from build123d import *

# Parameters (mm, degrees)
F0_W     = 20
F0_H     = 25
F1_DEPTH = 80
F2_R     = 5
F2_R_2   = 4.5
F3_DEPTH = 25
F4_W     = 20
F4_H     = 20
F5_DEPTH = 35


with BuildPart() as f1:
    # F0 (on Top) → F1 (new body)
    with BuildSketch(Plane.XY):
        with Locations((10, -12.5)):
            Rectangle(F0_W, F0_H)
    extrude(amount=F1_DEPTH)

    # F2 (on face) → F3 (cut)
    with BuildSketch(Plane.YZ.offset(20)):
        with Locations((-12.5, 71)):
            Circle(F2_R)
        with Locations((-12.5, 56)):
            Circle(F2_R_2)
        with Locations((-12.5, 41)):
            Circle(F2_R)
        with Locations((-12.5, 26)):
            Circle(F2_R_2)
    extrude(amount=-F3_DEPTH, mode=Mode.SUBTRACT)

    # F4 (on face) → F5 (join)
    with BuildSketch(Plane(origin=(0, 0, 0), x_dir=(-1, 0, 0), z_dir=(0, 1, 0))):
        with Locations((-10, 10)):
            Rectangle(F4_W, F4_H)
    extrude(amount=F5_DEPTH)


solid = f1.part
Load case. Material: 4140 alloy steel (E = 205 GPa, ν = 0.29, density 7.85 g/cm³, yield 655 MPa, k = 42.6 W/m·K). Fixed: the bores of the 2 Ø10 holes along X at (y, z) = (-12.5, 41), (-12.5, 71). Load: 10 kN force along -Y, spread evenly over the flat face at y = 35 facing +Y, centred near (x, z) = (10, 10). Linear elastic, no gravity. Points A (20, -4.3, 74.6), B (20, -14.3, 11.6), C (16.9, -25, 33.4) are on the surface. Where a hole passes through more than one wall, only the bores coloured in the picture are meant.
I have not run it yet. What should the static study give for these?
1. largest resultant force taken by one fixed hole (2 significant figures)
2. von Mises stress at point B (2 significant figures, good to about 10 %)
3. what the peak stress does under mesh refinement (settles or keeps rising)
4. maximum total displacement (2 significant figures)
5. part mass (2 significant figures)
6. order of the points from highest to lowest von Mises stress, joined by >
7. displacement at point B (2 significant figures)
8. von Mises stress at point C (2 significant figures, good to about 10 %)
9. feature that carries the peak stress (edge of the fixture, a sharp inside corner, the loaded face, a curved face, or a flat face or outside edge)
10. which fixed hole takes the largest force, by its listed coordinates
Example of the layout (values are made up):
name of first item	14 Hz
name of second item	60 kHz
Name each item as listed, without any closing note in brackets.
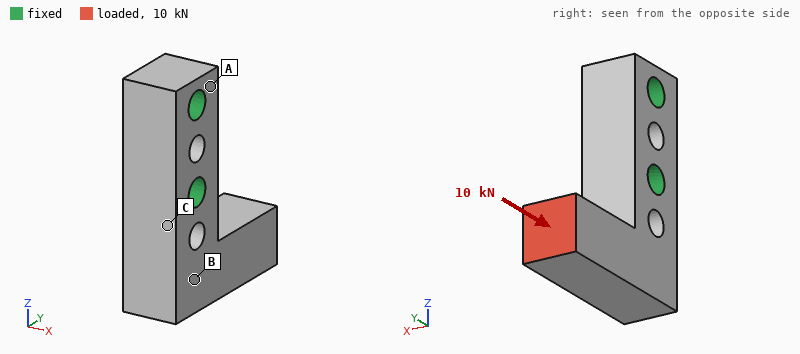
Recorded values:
largest resultant force taken by one fixed hole	13 kN
von Mises stress at point B	42 MPa
what the peak stress does under mesh refinement	keeps rising
maximum total displacement	86 µm
part mass	380 g
order of the points from highest to lowest von Mises stress, joined by >	C > B > A
displacement at point B	36 µm
von Mises stress at point C	140 MPa
feature that carries the peak stress	edge of the fixture
which fixed hole takes the largest force, by its listed coordinates	(-12.5, 41)
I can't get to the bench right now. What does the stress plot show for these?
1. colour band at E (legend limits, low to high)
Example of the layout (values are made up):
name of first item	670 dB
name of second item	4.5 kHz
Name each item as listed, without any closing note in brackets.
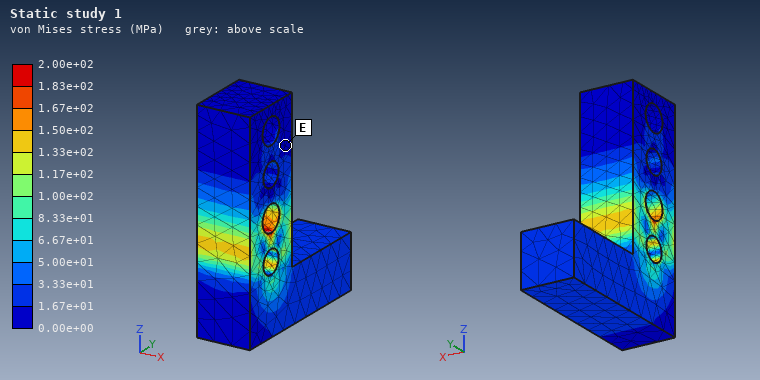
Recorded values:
colour band at E	0.00e+00 to 1.67e+01 MPa
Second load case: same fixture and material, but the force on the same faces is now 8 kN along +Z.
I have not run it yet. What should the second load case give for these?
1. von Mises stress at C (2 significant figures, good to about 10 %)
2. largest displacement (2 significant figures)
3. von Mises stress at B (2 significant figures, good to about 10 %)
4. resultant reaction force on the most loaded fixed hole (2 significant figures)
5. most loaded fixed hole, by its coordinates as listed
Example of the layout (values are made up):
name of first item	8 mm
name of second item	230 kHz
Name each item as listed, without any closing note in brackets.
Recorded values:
von Mises stress at C	180 MPa
largest displacement	0.22 mm
von Mises stress at B	110 MPa
resultant reaction force on the most loaded fixed hole	8.3 kN
most loaded fixed hole, by its coordinates as listed	(-12.5, 41)
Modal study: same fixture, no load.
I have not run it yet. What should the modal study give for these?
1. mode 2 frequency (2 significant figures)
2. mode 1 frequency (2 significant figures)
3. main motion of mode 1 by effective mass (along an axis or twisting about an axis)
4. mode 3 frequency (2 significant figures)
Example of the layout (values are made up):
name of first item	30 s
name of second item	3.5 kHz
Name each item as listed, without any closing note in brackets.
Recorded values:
mode 2 frequency	4000 Hz
mode 1 frequency	3500 Hz
main motion of mode 1 by effective mass	along X
mode 3 frequency	7600 Hz
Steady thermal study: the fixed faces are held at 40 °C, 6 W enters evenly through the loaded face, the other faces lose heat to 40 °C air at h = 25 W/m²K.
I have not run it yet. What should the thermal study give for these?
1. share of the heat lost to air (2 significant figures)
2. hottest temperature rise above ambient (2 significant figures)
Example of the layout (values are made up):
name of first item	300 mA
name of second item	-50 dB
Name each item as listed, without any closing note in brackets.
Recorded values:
share of the heat lost to air	24 %
hottest temperature rise above ambient	20 K
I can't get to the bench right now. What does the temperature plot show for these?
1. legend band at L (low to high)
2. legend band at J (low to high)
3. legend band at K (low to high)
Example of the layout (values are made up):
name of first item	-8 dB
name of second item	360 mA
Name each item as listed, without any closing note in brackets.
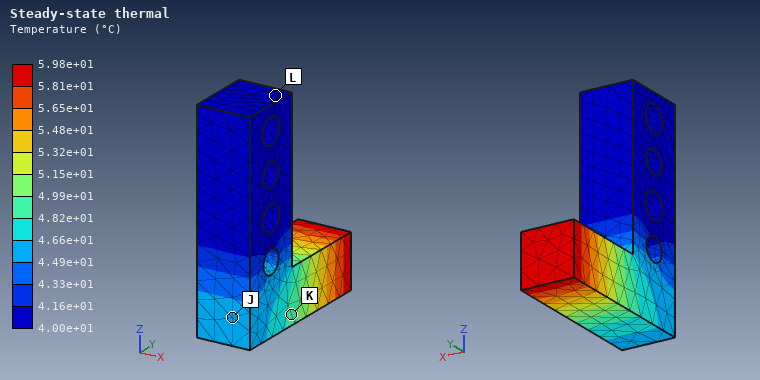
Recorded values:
legend band at L	4.00e+01 to 4.16e+01 °C
legend band at J	4.49e+01 to 4.66e+01 °C
legend band at K	4.82e+01 to 4.99e+01 °C
